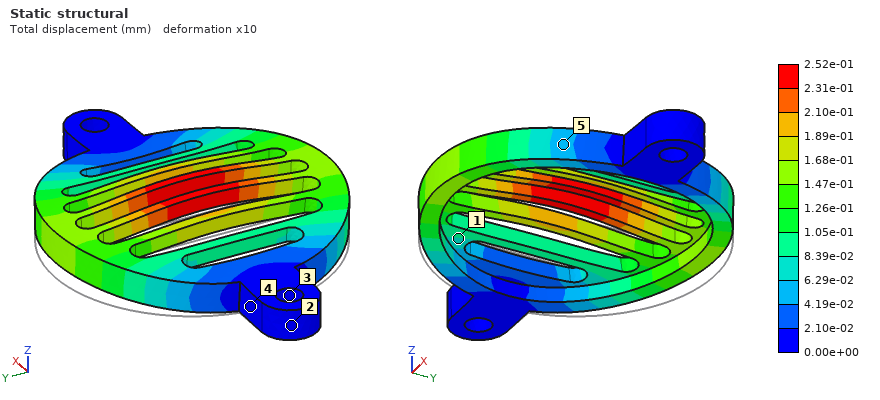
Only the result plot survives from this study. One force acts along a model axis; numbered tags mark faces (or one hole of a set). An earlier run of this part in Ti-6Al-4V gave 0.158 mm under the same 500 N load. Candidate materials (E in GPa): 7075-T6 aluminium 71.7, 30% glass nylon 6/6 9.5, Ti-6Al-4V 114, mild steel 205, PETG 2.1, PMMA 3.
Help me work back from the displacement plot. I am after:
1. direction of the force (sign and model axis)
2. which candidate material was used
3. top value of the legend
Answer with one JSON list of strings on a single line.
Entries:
["+Z", "7075-T6 aluminium", "2.52e-01 mm"]
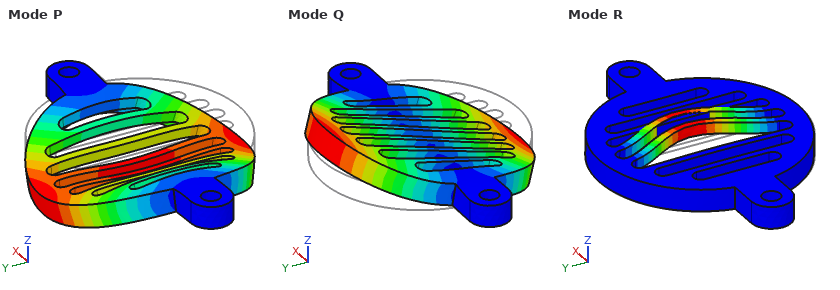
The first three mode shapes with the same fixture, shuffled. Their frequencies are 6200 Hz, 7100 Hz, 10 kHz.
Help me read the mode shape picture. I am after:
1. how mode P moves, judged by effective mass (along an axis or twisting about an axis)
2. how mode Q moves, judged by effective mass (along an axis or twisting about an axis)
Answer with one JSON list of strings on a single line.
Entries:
["along Z", "twisting about X"]
